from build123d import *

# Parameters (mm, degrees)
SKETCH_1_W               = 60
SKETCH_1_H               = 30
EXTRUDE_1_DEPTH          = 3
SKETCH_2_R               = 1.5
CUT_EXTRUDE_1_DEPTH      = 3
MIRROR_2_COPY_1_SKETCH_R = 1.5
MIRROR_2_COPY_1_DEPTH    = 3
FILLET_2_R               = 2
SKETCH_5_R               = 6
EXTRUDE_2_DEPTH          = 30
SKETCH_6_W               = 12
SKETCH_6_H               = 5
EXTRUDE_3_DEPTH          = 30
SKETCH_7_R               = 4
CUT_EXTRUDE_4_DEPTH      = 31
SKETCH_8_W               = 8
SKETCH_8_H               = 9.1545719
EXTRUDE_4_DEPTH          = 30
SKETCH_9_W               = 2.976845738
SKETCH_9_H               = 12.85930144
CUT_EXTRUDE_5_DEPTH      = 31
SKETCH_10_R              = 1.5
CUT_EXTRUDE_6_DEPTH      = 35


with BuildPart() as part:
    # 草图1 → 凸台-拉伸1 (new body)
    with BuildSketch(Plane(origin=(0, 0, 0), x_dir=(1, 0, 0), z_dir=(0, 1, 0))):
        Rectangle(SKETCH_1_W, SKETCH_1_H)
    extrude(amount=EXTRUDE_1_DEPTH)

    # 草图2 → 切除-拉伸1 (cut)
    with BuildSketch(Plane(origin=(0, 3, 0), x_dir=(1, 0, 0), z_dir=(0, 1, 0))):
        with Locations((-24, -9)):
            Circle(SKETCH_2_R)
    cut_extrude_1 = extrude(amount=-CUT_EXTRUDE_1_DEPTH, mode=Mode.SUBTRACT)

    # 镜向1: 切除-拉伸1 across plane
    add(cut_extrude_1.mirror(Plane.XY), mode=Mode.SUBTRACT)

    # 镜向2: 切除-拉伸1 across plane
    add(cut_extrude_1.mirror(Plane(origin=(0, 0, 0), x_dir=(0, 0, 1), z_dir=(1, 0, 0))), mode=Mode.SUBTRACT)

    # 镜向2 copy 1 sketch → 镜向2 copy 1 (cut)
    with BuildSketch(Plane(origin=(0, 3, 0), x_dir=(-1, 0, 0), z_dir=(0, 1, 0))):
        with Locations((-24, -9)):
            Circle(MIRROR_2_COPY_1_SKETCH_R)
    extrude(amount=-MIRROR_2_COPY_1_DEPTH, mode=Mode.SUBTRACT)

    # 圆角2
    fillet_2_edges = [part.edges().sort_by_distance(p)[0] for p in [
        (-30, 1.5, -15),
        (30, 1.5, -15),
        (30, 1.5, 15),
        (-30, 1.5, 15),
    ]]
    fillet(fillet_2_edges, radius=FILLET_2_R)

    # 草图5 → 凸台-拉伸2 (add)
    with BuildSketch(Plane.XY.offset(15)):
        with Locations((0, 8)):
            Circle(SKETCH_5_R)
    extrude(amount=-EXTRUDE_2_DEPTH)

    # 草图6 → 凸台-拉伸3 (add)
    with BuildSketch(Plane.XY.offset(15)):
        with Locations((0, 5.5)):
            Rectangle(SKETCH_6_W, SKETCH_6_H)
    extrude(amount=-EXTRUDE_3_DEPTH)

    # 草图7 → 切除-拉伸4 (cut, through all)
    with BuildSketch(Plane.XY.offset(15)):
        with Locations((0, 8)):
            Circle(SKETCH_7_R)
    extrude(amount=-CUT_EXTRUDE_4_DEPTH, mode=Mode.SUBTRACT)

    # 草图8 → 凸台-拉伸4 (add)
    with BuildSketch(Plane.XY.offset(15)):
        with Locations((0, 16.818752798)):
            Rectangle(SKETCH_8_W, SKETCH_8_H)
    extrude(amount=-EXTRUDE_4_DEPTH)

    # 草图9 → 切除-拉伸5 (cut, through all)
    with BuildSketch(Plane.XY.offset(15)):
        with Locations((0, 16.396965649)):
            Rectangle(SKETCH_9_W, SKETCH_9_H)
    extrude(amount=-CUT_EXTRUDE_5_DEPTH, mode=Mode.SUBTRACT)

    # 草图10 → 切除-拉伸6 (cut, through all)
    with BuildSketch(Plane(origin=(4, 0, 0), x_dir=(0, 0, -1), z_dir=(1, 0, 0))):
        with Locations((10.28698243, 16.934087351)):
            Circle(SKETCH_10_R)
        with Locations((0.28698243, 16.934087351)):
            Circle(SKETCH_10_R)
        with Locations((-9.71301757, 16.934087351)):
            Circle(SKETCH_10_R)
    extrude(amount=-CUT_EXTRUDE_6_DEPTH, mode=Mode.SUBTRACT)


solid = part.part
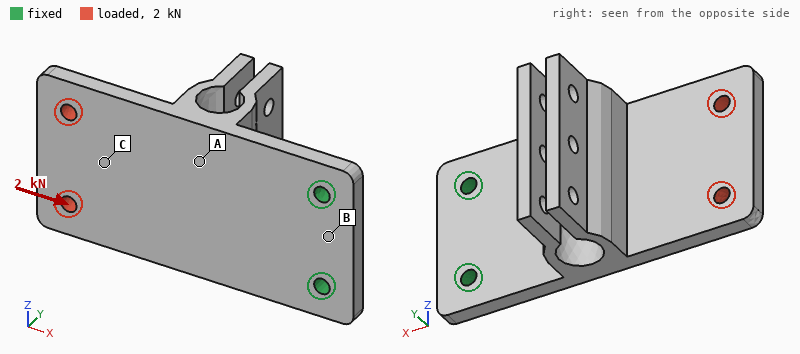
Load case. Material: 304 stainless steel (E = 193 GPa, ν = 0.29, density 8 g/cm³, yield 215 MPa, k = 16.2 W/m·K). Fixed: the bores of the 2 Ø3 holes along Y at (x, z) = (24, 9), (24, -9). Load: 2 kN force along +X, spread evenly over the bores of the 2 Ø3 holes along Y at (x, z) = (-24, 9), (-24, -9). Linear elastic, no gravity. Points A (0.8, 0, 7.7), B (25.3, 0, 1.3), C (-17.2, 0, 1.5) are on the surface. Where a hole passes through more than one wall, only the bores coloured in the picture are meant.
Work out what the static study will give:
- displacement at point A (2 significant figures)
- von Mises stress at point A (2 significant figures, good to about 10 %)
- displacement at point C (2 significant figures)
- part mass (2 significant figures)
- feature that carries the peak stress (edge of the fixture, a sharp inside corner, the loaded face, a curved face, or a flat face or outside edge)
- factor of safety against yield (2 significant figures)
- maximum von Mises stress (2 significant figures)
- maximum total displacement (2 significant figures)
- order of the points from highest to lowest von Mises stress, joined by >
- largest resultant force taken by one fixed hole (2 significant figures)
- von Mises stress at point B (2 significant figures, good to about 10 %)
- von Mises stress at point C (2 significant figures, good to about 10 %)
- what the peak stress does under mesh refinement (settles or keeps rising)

3.2 µm
28 MPa
8.1 µm
66 g
the loaded face
2.9
73 MPa
13 µm
A > C > B
1.0 kN
6.1 MPa
17 MPa
settles
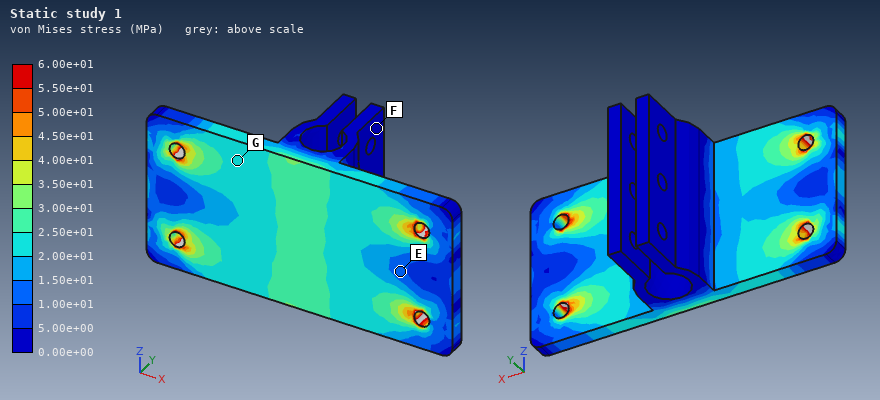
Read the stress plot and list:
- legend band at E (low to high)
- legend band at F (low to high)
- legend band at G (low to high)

1.00e+01 to 1.50e+01 MPa
0.00e+00 to 5.00e+00 MPa
2.00e+01 to 2.50e+01 MPa
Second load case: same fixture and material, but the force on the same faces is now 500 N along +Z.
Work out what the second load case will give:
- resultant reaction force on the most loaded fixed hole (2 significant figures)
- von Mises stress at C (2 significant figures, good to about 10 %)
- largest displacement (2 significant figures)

1.2 kN
13 MPa
24 µm
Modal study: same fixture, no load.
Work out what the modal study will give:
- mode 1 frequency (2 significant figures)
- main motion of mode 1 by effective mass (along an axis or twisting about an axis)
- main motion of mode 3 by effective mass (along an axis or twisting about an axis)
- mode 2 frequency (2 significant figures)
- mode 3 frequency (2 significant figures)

750 Hz
along Y
along Y
2600 Hz
4200 Hz
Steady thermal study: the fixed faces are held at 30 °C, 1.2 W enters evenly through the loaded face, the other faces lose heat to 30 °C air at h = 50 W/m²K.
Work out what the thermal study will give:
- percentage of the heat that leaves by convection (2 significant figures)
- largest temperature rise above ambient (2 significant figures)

90 %
14 K
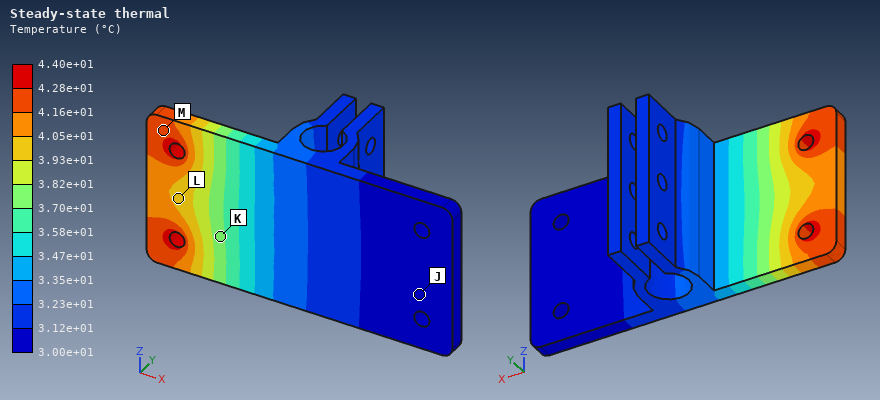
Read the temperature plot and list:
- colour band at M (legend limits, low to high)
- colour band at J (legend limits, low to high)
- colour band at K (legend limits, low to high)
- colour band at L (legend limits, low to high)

4.16e+01 to 4.28e+01 °C
3.00e+01 to 3.12e+01 °C
3.70e+01 to 3.82e+01 °C
3.93e+01 to 4.05e+01 °C
